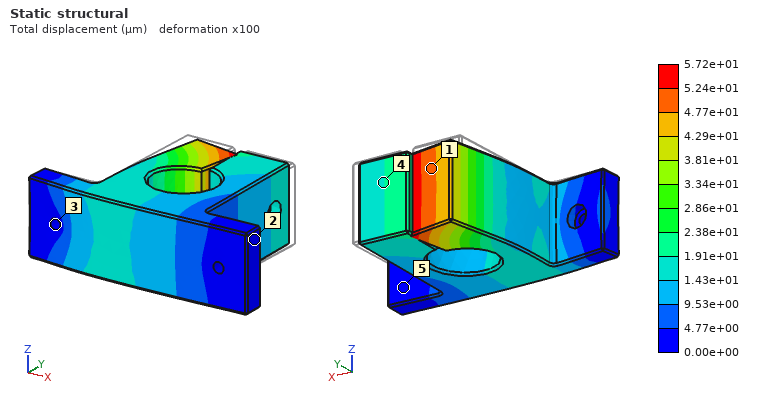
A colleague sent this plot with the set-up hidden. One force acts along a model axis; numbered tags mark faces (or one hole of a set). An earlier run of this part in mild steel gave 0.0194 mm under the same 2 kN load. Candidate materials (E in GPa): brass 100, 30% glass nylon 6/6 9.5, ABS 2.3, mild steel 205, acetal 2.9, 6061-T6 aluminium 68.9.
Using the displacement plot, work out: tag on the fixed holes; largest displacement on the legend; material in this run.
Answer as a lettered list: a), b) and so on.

a) 3
b) 5.72e+01 µm
c) 6061-T6 aluminium
